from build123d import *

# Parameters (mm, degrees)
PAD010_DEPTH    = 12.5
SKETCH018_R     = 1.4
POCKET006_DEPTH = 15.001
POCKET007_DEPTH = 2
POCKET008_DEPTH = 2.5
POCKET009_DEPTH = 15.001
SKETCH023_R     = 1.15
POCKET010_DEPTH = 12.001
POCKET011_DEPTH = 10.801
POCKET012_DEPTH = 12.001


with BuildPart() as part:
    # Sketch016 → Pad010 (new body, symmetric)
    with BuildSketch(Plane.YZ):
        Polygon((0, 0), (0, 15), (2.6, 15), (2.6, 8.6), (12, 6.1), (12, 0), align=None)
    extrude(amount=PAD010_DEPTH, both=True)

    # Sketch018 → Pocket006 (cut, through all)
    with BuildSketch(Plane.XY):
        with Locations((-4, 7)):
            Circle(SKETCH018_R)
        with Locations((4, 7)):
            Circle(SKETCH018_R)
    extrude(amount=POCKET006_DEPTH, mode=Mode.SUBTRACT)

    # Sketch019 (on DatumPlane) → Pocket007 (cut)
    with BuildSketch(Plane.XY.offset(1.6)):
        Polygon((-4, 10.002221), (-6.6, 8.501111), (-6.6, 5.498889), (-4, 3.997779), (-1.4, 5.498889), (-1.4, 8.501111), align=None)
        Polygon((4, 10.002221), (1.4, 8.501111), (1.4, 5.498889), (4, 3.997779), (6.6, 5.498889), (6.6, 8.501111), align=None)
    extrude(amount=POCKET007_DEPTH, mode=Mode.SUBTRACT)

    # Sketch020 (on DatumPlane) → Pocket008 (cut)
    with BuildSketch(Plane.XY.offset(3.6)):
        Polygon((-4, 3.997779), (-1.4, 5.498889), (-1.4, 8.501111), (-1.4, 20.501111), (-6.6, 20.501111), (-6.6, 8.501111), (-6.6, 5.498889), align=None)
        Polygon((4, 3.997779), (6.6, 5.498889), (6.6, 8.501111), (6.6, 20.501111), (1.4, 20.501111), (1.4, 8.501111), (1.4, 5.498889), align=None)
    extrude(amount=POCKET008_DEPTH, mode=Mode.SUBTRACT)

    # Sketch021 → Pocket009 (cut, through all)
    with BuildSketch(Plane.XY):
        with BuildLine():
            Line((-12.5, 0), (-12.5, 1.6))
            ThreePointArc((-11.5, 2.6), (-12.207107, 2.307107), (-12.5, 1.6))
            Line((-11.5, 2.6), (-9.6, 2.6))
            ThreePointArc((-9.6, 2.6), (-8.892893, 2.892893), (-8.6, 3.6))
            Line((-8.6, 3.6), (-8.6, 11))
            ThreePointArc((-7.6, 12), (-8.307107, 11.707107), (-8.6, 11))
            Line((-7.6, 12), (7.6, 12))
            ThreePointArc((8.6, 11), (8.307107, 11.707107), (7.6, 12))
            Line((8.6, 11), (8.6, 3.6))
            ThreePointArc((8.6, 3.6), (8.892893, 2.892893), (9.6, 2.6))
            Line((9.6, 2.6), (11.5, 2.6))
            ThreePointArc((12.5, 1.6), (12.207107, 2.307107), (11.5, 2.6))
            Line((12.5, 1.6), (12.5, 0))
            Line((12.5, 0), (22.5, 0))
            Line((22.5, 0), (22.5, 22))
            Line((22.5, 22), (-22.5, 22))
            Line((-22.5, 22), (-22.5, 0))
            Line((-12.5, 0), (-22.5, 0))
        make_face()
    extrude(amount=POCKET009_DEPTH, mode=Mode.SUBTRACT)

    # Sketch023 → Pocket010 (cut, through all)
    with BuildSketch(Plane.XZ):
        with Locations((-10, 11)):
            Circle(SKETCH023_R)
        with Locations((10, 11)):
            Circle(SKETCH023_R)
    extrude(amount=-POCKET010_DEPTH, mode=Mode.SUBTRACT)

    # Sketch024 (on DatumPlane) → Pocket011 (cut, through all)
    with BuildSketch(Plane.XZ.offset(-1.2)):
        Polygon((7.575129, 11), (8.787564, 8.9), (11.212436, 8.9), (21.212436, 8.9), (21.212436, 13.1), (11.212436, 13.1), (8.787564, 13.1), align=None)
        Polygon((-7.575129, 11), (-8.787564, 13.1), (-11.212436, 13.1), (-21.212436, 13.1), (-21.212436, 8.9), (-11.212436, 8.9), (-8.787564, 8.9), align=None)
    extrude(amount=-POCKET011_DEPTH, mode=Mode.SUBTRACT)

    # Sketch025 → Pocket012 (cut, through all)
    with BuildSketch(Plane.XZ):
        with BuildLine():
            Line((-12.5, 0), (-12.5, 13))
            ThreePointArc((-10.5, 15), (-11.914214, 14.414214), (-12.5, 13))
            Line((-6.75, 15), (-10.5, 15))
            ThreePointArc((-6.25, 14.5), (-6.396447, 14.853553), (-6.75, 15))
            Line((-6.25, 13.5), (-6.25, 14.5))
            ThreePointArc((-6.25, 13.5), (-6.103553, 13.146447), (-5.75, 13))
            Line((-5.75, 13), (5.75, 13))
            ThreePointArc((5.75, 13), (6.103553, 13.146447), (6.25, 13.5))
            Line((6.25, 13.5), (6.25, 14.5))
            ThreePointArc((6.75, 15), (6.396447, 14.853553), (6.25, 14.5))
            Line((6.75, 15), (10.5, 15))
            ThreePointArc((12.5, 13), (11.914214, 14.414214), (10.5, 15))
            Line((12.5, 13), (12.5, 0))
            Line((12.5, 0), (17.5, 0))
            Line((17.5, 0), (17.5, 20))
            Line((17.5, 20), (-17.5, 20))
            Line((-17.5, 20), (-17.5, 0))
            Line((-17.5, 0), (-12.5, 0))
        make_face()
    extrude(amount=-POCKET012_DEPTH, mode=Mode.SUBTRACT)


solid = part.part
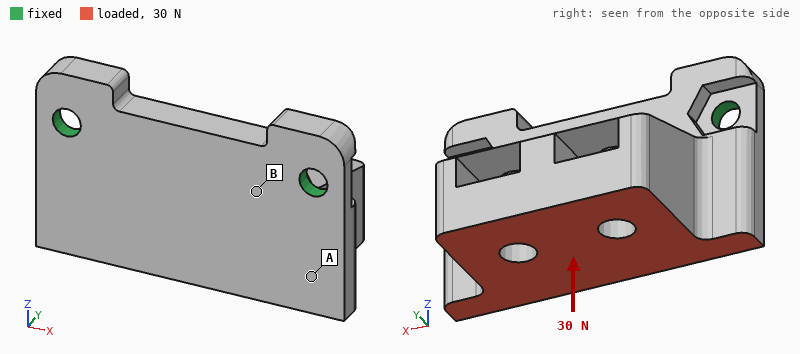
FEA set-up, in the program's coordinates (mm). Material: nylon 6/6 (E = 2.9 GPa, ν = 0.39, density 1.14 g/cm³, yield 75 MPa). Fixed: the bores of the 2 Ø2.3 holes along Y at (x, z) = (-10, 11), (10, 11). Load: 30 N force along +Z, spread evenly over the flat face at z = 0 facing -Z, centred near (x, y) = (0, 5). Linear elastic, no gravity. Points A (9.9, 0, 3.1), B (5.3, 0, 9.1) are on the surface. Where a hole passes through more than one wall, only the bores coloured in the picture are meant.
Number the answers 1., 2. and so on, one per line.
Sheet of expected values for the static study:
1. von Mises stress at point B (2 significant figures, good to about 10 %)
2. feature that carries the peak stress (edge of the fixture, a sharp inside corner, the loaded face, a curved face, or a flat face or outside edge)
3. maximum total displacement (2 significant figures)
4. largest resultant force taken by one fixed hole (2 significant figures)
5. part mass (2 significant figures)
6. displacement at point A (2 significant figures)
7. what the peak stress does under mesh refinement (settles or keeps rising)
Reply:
1. 5.1 MPa
2. edge of the fixture
3. 0.30 mm
4. 17 N
5. 2.0 g
6. 0.13 mm
7. keeps rising
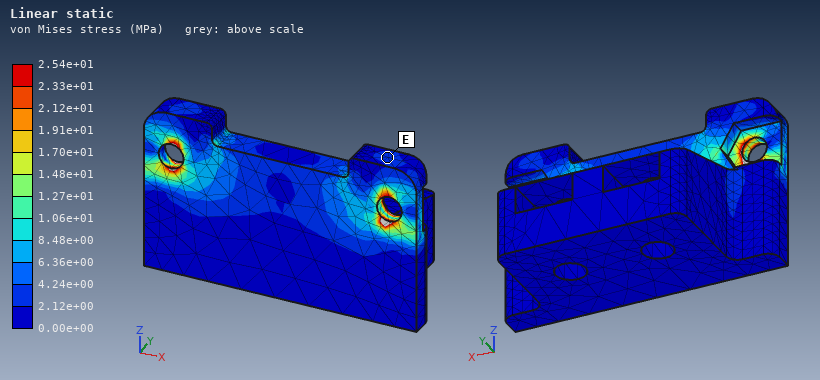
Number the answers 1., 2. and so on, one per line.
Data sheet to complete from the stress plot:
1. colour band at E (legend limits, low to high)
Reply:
1. 2.12e+00 to 4.24e+00 MPa
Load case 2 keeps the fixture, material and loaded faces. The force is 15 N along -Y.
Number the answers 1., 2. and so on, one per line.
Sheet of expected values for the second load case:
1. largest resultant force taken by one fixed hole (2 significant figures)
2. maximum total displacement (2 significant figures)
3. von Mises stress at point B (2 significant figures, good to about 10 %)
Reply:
1. 7.5 N
2. 0.31 mm
3. 5.3 MPa
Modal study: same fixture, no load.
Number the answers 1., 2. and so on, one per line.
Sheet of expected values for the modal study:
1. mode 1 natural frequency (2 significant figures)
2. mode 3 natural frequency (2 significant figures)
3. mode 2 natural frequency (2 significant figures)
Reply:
1. 1300 Hz
2. 7800 Hz
3. 5900 Hz
